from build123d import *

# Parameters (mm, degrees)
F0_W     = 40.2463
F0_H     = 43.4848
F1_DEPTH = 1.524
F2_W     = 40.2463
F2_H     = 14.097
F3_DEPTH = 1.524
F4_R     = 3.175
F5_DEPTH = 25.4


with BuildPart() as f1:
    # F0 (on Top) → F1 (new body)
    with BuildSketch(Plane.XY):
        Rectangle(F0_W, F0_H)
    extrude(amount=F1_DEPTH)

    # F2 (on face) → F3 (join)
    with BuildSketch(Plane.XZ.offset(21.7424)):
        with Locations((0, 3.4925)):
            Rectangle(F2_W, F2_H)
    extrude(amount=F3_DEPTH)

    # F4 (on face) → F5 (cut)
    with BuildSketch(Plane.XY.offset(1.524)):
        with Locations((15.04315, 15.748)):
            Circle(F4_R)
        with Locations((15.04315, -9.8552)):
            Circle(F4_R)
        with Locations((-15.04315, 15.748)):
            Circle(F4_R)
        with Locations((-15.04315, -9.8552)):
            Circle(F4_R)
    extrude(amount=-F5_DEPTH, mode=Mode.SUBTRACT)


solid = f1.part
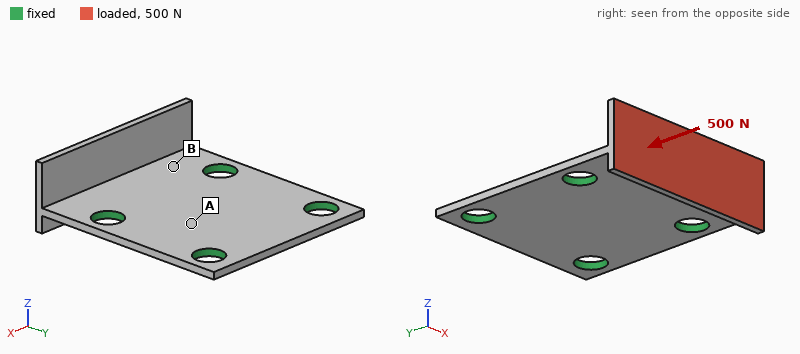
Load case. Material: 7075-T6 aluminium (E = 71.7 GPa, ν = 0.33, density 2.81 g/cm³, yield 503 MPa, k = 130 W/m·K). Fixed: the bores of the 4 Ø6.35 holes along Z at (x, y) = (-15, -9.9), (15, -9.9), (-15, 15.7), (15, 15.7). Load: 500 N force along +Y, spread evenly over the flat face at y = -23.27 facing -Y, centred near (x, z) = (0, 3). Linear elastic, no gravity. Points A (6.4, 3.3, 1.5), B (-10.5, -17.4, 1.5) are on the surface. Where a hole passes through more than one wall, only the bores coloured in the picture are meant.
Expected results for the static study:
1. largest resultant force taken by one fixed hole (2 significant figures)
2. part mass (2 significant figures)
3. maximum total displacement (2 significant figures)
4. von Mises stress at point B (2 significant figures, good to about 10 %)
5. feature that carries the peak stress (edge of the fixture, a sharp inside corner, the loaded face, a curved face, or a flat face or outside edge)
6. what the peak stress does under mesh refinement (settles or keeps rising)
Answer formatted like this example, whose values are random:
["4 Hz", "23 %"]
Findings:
["220 N", "9.4 g", "0.22 mm", "88 MPa", "edge of the fixture", "keeps rising"]
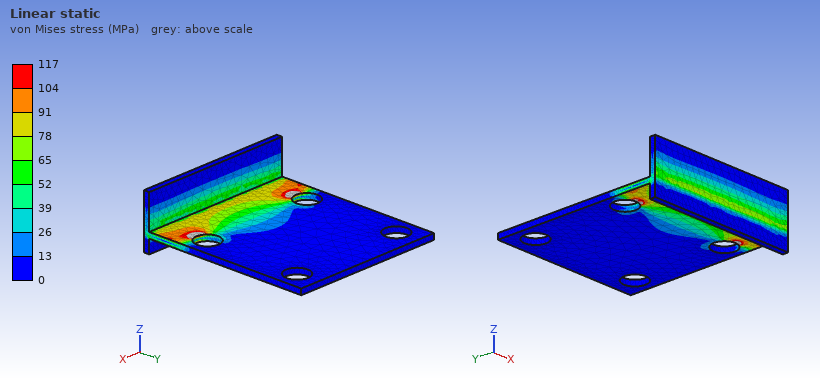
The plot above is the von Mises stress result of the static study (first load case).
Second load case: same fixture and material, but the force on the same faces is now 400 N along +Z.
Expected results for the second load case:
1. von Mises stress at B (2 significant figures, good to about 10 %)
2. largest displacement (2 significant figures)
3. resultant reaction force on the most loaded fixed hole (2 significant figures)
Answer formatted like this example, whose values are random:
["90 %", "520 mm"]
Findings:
["140 MPa", "0.40 mm", "210 N"]
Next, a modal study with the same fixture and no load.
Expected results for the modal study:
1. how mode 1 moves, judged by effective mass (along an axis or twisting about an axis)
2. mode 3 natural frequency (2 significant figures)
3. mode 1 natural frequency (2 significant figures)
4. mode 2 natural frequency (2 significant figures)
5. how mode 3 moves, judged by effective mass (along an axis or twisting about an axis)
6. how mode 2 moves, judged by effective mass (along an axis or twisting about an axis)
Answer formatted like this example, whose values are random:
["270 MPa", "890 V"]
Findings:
["along Z", "9900 Hz", "3600 Hz", "5800 Hz", "along Z", "twisting about Y"]
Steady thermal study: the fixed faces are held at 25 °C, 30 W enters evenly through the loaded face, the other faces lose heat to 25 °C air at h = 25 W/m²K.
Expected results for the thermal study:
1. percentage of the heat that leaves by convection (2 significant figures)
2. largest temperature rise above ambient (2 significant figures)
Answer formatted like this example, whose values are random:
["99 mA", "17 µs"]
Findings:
["5.2 %", "57 K"]
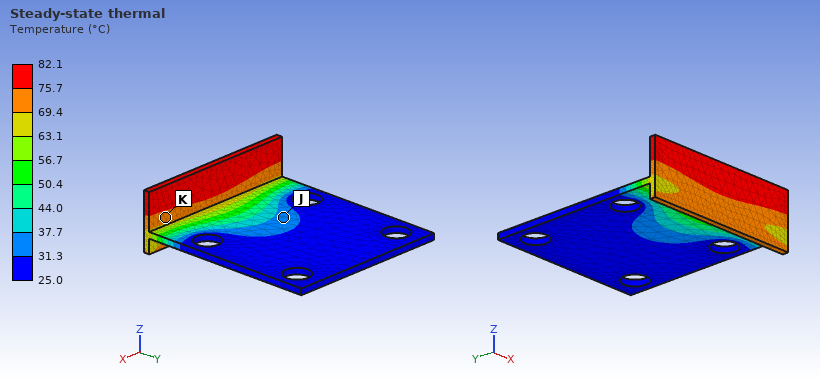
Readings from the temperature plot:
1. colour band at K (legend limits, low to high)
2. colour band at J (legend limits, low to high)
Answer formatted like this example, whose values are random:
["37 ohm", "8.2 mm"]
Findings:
["69.4 to 75.7 °C", "31.3 to 37.7 °C"]
